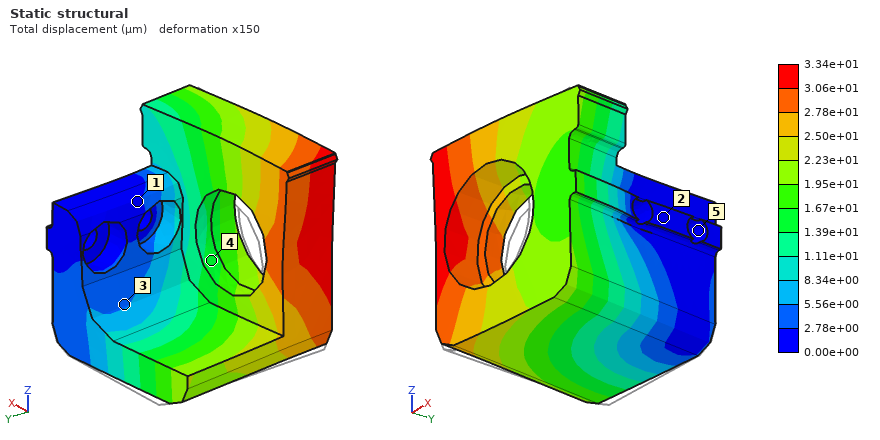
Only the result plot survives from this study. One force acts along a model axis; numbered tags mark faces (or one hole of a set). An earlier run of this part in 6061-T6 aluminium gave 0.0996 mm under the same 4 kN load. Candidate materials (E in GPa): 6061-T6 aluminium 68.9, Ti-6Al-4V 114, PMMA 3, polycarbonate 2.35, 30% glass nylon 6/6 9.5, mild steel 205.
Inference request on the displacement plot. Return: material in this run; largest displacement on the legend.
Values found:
mild steel
3.34e+01 µm
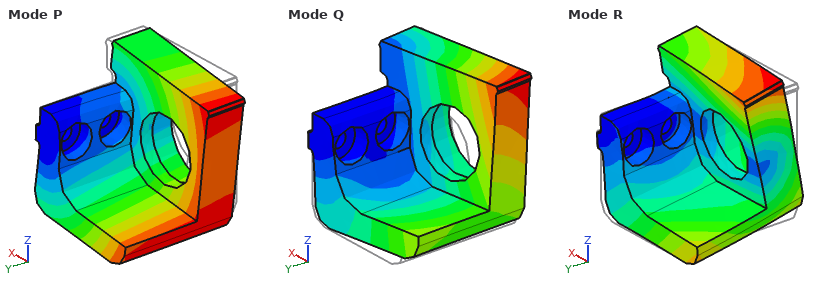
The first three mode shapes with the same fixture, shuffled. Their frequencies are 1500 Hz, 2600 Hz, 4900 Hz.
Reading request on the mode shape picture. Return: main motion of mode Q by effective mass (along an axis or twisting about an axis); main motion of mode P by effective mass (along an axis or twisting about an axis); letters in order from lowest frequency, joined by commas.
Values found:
along Y
along Z
P, Q, R
